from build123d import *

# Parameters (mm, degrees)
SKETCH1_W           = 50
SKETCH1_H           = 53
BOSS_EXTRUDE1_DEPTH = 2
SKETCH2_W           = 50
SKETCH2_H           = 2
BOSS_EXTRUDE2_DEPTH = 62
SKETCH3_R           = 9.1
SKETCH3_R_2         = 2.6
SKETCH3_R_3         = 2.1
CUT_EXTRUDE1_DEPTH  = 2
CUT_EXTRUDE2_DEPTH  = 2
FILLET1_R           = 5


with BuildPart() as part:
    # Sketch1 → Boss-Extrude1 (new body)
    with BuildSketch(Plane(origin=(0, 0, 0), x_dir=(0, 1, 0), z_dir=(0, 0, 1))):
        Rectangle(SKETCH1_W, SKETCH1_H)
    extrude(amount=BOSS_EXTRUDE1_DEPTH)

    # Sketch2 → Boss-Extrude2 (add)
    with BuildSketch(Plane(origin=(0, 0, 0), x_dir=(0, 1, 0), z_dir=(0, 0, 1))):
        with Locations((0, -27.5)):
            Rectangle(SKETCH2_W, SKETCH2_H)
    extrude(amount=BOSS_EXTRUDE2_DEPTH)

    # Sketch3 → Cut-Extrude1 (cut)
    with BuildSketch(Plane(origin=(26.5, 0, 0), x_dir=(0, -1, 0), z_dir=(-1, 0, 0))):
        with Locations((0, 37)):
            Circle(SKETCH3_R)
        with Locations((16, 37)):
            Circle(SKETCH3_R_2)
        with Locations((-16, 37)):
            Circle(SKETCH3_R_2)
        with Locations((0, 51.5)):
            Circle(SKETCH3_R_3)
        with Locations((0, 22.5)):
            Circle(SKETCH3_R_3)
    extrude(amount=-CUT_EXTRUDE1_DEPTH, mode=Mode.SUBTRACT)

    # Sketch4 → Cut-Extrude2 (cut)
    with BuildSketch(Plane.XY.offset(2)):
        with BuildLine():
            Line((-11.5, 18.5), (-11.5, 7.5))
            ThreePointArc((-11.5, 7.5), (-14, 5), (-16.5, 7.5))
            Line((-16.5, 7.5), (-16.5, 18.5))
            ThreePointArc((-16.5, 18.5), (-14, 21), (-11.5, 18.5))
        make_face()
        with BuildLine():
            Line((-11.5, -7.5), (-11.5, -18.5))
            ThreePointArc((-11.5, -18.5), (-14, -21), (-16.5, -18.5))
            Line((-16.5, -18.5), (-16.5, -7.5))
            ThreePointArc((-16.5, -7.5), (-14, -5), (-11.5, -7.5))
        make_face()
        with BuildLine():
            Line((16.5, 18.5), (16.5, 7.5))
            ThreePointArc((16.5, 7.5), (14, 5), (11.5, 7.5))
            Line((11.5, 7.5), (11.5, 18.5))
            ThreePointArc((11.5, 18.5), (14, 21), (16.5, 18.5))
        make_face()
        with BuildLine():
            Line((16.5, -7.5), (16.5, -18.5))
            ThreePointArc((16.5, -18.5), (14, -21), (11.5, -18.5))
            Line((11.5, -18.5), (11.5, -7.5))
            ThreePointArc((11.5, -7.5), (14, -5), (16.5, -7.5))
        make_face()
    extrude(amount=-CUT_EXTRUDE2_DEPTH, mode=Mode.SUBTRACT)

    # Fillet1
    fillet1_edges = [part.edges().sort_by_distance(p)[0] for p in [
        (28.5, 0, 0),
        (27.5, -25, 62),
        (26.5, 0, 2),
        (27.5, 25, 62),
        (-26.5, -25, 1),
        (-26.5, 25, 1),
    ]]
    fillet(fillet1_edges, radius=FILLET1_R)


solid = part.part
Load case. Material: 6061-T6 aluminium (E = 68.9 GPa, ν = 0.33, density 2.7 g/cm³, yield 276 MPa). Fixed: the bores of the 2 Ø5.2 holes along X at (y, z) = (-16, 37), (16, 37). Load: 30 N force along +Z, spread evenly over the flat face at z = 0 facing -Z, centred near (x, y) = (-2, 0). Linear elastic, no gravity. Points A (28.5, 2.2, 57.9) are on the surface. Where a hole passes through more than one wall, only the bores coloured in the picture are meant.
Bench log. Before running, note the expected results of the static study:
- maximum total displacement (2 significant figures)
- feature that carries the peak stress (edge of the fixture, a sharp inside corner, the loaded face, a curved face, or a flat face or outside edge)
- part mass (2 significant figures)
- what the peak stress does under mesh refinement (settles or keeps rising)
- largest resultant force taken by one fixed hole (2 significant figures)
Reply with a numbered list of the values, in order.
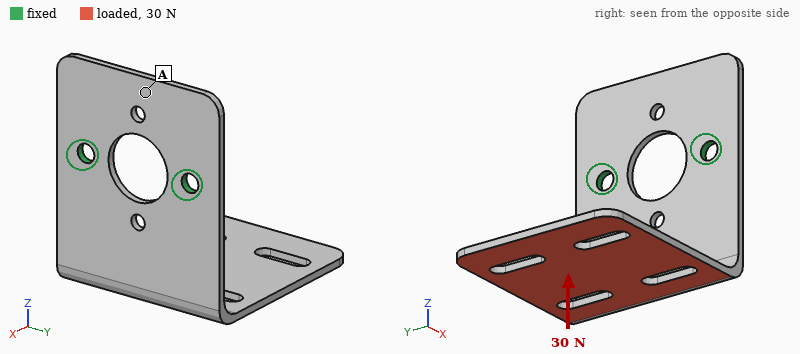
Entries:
1. 1.1 mm
2. edge of the fixture
3. 28 g
4. keeps rising
5. 16 N
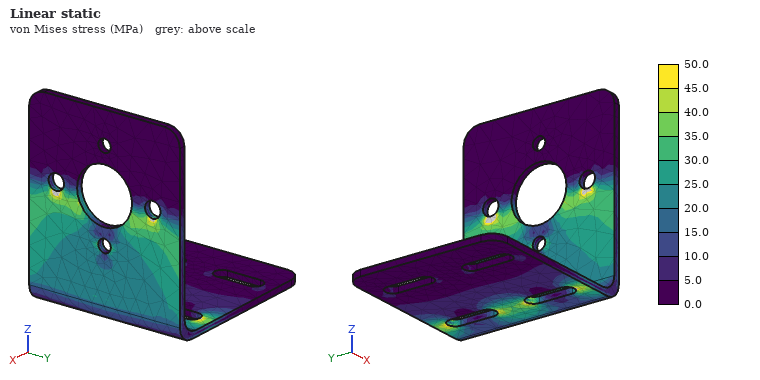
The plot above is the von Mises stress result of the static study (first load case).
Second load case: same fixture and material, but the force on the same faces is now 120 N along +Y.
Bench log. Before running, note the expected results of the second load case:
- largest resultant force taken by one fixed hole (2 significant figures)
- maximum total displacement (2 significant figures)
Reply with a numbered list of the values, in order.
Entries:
1. 160 N
2. 1.0 mm
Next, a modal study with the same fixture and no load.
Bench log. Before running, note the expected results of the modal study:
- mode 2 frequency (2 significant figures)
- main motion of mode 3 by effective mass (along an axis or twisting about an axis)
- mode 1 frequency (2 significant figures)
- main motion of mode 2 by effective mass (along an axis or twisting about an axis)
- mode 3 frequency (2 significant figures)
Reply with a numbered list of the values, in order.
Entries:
1. 560 Hz
2. along X
3. 270 Hz
4. along Y
5. 780 Hz
